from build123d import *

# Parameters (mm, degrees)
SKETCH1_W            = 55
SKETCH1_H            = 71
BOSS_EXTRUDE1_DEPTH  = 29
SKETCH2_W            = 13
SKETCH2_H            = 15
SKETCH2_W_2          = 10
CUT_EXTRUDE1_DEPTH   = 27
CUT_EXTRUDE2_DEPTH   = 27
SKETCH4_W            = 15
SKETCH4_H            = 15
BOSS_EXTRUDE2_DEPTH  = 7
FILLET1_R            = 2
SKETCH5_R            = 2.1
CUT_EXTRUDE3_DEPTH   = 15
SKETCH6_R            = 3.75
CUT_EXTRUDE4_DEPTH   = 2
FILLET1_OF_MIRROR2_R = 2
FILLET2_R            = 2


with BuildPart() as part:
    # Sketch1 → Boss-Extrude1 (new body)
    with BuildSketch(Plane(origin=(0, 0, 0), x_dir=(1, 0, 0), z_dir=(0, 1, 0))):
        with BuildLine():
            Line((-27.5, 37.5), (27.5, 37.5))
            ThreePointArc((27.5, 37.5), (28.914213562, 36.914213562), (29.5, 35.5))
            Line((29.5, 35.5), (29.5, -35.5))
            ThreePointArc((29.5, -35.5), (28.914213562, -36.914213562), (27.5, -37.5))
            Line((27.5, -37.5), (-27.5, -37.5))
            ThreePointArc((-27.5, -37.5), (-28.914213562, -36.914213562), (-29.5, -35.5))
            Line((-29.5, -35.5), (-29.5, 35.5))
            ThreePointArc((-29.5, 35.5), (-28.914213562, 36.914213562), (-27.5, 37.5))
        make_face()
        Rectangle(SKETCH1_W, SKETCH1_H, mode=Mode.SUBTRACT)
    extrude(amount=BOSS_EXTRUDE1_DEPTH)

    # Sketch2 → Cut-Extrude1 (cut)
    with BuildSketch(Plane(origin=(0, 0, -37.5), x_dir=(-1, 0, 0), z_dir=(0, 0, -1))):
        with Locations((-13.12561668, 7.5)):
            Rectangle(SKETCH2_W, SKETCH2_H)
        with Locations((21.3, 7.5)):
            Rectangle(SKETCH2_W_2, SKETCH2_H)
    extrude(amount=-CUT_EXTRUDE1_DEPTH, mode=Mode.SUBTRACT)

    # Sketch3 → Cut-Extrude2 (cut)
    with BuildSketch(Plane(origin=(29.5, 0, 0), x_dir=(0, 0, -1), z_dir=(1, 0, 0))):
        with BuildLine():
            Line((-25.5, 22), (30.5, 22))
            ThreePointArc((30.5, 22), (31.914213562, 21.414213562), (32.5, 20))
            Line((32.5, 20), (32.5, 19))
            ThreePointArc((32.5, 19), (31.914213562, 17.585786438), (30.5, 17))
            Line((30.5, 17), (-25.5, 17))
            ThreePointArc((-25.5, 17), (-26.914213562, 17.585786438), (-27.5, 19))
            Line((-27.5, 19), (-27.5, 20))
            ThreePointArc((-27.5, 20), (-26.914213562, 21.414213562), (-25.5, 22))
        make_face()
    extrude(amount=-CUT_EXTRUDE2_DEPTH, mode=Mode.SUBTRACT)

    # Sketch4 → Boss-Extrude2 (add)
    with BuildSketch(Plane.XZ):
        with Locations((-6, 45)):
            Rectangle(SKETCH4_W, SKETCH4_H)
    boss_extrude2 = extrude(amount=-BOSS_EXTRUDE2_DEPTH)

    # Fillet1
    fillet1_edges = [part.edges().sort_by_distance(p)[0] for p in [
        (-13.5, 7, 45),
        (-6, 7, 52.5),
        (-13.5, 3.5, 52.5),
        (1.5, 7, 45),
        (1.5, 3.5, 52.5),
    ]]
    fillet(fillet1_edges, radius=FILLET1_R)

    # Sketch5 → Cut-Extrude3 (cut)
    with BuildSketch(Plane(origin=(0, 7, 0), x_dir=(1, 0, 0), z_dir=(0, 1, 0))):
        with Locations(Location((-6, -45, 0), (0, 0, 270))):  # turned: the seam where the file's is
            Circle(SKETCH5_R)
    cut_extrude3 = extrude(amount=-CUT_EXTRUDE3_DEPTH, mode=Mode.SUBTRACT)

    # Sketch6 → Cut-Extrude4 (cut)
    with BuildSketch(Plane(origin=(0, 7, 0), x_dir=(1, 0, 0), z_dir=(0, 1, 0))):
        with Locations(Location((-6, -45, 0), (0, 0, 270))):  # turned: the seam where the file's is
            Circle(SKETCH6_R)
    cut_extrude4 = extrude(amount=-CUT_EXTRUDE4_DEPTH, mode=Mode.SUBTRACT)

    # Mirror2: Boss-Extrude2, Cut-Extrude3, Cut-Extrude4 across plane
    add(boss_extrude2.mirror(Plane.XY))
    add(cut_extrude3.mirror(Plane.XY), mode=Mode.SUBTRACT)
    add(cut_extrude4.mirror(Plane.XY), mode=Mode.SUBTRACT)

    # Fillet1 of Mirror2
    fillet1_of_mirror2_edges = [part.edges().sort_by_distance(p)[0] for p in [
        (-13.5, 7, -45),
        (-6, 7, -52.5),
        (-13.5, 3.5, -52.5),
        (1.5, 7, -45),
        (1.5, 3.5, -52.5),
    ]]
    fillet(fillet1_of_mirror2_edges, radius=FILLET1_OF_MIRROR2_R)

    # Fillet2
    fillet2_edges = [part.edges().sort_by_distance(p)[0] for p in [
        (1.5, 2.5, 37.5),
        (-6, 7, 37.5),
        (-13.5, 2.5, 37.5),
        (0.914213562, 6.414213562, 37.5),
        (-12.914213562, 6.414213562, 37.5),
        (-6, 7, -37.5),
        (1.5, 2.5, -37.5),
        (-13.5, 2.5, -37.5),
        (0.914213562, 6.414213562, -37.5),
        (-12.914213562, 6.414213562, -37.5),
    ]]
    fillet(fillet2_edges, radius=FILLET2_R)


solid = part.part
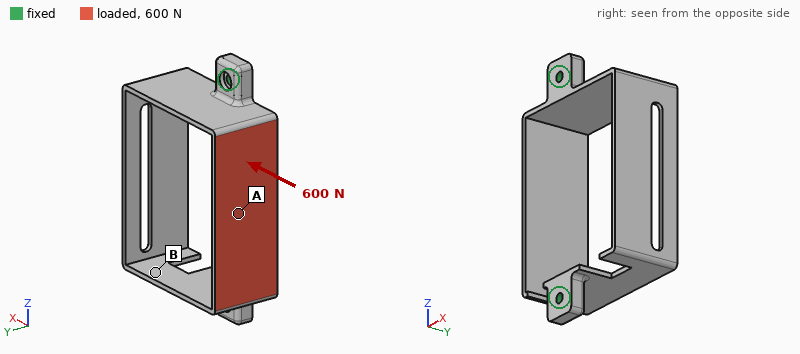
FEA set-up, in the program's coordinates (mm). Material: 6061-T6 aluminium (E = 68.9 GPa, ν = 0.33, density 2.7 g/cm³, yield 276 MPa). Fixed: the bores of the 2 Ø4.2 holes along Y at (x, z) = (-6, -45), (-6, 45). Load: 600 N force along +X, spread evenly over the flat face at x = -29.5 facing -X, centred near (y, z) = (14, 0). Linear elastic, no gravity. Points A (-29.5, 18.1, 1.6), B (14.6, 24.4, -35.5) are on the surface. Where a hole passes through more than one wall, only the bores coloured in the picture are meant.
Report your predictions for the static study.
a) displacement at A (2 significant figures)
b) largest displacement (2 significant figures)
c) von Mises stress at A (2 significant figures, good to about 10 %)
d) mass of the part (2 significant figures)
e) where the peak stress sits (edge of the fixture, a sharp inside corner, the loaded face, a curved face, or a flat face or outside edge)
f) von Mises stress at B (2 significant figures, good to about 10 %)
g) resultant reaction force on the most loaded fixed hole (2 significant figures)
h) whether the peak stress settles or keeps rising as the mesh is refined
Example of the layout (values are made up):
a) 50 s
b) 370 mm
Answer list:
a) 0.87 mm
b) 0.98 mm
c) 130 MPa
d) 45 g
e) a sharp inside corner
f) 18 MPa
g) 360 N
h) keeps rising
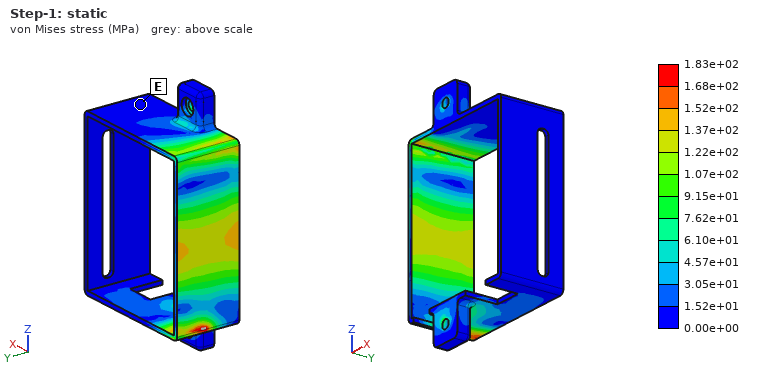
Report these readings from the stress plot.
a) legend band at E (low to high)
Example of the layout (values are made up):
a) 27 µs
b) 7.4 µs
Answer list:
a) 0.00e+00 to 1.52e+01 MPa
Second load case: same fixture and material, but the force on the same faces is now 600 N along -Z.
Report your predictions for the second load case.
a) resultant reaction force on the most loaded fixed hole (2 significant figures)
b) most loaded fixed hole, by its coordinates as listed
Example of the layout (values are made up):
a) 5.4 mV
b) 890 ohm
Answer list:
a) 430 N
b) (-6, 45)
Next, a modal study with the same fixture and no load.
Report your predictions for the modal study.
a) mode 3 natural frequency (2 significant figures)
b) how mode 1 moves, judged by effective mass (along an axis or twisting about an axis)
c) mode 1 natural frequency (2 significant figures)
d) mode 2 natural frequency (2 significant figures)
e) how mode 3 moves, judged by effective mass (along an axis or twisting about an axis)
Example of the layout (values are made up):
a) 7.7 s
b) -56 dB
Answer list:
a) 1400 Hz
b) along Z
c) 920 Hz
d) 1300 Hz
e) along X
